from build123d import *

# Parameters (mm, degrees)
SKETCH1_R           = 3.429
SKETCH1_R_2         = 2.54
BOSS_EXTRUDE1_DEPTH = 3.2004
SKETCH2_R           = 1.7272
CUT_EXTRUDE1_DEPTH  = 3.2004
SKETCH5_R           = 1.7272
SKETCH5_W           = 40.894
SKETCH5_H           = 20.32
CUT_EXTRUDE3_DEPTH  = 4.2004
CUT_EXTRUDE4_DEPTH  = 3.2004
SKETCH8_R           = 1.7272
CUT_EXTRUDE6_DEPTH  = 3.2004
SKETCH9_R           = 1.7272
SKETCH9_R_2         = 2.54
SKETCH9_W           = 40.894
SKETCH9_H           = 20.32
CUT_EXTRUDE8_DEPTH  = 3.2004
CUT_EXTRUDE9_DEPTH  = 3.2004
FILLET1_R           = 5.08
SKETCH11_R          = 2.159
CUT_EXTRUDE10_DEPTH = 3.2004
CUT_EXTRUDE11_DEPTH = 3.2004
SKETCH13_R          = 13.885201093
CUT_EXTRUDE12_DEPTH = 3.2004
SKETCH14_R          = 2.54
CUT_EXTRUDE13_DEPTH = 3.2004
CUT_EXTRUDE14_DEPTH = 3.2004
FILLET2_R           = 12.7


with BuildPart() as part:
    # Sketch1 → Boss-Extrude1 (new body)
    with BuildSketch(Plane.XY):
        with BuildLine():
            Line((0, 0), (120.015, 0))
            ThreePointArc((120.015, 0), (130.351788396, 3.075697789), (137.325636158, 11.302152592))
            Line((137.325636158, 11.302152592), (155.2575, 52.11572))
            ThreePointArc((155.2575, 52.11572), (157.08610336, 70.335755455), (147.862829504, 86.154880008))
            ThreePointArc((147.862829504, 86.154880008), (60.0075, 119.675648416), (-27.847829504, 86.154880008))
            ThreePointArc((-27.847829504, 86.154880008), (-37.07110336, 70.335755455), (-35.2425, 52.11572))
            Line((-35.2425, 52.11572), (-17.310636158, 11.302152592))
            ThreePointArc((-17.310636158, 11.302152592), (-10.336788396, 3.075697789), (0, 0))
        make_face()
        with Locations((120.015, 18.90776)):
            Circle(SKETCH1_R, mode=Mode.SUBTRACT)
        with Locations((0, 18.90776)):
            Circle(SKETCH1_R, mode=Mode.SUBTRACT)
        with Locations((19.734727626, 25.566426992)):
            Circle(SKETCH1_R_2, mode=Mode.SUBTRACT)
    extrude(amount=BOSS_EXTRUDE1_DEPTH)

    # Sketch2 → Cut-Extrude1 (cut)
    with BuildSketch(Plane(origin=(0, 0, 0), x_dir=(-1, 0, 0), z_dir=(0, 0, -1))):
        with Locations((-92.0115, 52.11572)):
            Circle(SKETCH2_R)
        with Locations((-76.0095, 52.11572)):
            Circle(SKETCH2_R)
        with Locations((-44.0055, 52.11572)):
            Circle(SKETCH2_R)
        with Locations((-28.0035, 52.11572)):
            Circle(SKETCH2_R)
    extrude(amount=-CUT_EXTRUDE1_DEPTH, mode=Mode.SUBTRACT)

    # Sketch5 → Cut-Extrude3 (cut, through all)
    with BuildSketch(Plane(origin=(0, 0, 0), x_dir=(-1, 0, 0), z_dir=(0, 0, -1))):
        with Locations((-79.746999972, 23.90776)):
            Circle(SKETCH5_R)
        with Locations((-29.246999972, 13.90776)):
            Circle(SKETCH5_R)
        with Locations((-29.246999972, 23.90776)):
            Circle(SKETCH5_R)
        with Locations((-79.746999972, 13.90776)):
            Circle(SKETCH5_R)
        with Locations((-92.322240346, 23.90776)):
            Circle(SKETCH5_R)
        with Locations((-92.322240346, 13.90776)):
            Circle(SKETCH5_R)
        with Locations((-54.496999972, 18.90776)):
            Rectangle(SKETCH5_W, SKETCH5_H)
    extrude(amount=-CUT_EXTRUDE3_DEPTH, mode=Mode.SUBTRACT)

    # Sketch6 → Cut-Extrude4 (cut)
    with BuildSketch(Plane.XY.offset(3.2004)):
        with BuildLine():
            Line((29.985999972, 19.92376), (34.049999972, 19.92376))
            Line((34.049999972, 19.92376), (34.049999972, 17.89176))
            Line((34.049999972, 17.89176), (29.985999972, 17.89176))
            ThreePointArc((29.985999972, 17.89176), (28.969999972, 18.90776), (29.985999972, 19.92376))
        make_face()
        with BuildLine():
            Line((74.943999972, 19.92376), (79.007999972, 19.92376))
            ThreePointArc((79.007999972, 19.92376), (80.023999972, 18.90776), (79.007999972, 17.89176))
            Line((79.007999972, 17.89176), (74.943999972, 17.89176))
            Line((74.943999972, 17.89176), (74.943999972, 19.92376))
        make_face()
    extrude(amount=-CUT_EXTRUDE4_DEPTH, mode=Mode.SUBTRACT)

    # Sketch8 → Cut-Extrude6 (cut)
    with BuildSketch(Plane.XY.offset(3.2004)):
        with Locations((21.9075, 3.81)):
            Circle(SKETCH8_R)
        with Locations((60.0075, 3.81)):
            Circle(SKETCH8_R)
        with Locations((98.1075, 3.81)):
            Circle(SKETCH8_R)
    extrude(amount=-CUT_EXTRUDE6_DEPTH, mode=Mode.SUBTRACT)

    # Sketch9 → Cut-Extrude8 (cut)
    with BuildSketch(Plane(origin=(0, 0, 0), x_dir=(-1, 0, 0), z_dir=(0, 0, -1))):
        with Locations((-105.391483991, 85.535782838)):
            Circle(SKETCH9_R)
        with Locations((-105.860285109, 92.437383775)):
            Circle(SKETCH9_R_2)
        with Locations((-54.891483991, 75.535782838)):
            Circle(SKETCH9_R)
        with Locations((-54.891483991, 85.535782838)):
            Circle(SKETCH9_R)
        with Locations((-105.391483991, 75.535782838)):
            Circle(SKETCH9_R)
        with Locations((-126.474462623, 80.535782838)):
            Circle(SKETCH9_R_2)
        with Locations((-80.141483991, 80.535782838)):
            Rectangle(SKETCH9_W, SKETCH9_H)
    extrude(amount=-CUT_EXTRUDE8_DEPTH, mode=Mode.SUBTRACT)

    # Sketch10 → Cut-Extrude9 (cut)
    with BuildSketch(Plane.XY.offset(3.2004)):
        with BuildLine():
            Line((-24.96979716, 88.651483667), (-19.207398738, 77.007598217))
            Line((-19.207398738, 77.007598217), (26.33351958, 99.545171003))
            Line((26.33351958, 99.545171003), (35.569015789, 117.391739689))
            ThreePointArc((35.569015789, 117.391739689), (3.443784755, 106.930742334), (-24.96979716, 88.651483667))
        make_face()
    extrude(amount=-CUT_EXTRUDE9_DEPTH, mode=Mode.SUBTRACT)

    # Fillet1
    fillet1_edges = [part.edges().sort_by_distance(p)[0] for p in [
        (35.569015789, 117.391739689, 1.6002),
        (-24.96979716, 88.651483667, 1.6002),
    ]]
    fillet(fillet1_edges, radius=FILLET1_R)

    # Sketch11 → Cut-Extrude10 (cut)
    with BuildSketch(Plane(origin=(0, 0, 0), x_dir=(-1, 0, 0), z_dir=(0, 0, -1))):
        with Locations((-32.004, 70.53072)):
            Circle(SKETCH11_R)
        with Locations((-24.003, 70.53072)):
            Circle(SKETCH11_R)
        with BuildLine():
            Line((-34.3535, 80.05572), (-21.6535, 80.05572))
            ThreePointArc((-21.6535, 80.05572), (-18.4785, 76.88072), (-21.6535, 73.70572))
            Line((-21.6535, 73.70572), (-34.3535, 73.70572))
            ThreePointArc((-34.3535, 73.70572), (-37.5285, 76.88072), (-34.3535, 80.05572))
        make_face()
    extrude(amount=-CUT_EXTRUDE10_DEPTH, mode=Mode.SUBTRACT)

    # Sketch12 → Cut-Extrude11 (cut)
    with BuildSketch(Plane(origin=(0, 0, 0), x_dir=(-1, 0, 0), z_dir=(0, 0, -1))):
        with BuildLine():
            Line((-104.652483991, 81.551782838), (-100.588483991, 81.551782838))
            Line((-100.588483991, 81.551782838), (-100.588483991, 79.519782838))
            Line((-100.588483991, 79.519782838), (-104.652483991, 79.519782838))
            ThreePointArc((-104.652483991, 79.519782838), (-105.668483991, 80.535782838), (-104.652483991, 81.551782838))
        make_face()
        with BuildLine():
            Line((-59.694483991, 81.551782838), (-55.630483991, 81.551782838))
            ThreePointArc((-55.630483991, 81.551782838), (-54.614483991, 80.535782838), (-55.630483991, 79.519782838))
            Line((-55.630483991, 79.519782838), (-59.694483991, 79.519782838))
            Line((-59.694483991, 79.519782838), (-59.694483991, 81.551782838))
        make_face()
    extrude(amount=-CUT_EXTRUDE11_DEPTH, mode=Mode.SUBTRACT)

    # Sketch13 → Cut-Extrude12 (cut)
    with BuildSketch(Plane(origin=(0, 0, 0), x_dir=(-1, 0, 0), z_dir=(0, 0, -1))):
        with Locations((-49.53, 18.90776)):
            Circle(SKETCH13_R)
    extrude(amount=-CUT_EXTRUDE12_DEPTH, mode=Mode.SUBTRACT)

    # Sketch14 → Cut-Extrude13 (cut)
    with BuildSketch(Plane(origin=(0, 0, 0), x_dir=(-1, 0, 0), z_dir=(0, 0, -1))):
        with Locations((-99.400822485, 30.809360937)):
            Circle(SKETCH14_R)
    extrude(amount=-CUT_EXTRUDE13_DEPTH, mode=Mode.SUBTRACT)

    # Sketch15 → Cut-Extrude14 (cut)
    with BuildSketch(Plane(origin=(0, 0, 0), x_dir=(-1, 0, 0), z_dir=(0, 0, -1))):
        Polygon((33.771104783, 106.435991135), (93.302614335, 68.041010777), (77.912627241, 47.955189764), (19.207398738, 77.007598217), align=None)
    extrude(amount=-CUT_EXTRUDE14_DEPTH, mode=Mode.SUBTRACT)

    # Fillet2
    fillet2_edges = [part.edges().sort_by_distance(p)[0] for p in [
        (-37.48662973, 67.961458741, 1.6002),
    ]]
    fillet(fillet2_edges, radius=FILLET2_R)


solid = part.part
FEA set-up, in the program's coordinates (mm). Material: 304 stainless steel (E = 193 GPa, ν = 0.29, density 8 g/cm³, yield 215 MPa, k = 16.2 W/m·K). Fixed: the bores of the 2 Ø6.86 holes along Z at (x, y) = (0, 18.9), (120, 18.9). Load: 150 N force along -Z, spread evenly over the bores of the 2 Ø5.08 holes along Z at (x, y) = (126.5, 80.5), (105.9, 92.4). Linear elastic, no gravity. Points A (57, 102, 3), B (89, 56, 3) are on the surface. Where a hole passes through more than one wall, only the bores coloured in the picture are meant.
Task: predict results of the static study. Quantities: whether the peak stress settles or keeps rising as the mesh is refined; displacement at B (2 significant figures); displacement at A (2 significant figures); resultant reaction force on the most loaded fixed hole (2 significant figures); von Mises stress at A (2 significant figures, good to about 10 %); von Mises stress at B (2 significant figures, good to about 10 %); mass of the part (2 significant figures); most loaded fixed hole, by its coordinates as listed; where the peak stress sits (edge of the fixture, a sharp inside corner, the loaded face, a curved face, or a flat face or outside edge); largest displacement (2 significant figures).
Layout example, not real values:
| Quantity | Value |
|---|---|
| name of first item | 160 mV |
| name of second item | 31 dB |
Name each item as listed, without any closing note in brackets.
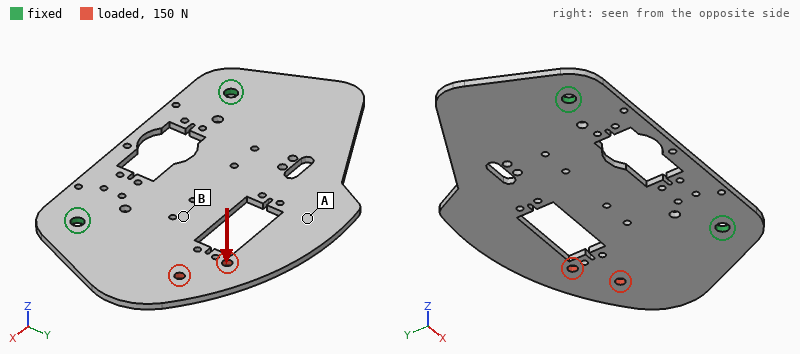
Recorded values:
| Quantity | Value |
|---|---|
| whether the peak stress settles or keeps rising as the mesh is refined | keeps rising |
| displacement at B | 0.13 mm |
| displacement at A | 0.33 mm |
| resultant reaction force on the most loaded fixed hole | 140 N |
| von Mises stress at A | 11 MPa |
| von Mises stress at B | 25 MPa |
| mass of the part | 410 g |
| most loaded fixed hole, by its coordinates as listed | (120, 18.9) |
| where the peak stress sits | edge of the fixture |
| largest displacement | 0.52 mm |
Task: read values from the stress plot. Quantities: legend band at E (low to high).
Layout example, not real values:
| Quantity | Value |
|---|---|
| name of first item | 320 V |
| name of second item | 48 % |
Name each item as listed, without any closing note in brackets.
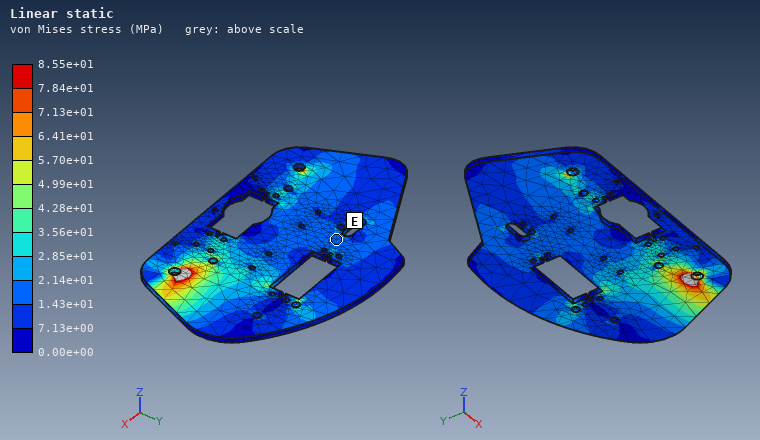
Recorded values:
| Quantity | Value |
|---|---|
| legend band at E | 1.43e+01 to 2.14e+01 MPa |
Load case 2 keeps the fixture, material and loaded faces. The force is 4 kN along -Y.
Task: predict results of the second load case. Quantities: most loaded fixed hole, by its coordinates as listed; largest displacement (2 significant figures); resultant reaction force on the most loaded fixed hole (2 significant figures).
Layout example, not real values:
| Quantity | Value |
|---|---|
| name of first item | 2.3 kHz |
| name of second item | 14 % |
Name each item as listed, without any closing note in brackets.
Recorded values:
| Quantity | Value |
|---|---|
| most loaded fixed hole, by its coordinates as listed | (120, 18.9) |
| largest displacement | 16 µm |
| resultant reaction force on the most loaded fixed hole | 3.8 kN |
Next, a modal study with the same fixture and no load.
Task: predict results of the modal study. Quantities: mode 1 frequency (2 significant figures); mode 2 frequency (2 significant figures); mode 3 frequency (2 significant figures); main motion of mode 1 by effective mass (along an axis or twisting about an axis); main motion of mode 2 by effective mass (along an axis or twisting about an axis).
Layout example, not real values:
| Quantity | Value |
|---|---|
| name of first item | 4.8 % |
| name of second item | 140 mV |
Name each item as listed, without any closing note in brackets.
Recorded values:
| Quantity | Value |
|---|---|
| mode 1 frequency | 270 Hz |
| mode 2 frequency | 570 Hz |
| mode 3 frequency | 920 Hz |
| main motion of mode 1 by effective mass | along Z |
| main motion of mode 2 by effective mass | twisting about Y |
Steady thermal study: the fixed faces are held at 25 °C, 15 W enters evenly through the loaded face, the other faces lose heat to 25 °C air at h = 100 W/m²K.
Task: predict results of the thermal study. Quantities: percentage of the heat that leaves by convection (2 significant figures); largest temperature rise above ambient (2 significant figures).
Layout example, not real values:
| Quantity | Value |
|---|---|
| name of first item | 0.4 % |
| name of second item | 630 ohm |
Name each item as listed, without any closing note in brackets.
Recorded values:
| Quantity | Value |
|---|---|
| percentage of the heat that leaves by convection | 99 % |
| largest temperature rise above ambient | 68 K |
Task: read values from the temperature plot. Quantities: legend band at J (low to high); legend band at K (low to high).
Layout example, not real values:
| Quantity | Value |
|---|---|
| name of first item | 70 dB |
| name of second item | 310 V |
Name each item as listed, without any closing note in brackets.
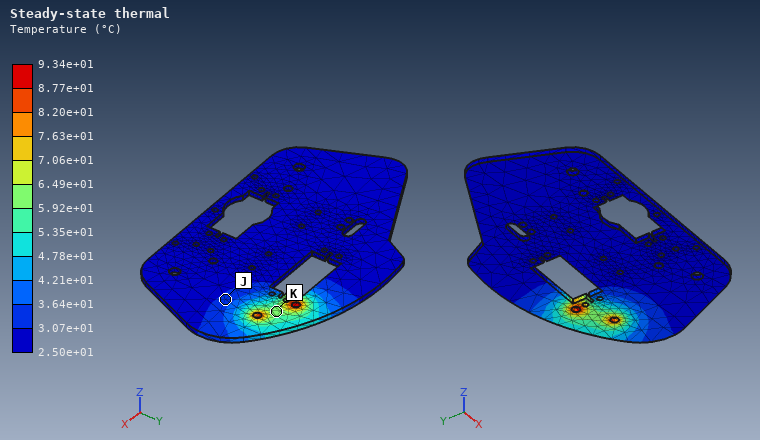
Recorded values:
| Quantity | Value |
|---|---|
| legend band at J | 3.07e+01 to 3.64e+01 °C |
| legend band at K | 5.92e+01 to 6.49e+01 °C |
